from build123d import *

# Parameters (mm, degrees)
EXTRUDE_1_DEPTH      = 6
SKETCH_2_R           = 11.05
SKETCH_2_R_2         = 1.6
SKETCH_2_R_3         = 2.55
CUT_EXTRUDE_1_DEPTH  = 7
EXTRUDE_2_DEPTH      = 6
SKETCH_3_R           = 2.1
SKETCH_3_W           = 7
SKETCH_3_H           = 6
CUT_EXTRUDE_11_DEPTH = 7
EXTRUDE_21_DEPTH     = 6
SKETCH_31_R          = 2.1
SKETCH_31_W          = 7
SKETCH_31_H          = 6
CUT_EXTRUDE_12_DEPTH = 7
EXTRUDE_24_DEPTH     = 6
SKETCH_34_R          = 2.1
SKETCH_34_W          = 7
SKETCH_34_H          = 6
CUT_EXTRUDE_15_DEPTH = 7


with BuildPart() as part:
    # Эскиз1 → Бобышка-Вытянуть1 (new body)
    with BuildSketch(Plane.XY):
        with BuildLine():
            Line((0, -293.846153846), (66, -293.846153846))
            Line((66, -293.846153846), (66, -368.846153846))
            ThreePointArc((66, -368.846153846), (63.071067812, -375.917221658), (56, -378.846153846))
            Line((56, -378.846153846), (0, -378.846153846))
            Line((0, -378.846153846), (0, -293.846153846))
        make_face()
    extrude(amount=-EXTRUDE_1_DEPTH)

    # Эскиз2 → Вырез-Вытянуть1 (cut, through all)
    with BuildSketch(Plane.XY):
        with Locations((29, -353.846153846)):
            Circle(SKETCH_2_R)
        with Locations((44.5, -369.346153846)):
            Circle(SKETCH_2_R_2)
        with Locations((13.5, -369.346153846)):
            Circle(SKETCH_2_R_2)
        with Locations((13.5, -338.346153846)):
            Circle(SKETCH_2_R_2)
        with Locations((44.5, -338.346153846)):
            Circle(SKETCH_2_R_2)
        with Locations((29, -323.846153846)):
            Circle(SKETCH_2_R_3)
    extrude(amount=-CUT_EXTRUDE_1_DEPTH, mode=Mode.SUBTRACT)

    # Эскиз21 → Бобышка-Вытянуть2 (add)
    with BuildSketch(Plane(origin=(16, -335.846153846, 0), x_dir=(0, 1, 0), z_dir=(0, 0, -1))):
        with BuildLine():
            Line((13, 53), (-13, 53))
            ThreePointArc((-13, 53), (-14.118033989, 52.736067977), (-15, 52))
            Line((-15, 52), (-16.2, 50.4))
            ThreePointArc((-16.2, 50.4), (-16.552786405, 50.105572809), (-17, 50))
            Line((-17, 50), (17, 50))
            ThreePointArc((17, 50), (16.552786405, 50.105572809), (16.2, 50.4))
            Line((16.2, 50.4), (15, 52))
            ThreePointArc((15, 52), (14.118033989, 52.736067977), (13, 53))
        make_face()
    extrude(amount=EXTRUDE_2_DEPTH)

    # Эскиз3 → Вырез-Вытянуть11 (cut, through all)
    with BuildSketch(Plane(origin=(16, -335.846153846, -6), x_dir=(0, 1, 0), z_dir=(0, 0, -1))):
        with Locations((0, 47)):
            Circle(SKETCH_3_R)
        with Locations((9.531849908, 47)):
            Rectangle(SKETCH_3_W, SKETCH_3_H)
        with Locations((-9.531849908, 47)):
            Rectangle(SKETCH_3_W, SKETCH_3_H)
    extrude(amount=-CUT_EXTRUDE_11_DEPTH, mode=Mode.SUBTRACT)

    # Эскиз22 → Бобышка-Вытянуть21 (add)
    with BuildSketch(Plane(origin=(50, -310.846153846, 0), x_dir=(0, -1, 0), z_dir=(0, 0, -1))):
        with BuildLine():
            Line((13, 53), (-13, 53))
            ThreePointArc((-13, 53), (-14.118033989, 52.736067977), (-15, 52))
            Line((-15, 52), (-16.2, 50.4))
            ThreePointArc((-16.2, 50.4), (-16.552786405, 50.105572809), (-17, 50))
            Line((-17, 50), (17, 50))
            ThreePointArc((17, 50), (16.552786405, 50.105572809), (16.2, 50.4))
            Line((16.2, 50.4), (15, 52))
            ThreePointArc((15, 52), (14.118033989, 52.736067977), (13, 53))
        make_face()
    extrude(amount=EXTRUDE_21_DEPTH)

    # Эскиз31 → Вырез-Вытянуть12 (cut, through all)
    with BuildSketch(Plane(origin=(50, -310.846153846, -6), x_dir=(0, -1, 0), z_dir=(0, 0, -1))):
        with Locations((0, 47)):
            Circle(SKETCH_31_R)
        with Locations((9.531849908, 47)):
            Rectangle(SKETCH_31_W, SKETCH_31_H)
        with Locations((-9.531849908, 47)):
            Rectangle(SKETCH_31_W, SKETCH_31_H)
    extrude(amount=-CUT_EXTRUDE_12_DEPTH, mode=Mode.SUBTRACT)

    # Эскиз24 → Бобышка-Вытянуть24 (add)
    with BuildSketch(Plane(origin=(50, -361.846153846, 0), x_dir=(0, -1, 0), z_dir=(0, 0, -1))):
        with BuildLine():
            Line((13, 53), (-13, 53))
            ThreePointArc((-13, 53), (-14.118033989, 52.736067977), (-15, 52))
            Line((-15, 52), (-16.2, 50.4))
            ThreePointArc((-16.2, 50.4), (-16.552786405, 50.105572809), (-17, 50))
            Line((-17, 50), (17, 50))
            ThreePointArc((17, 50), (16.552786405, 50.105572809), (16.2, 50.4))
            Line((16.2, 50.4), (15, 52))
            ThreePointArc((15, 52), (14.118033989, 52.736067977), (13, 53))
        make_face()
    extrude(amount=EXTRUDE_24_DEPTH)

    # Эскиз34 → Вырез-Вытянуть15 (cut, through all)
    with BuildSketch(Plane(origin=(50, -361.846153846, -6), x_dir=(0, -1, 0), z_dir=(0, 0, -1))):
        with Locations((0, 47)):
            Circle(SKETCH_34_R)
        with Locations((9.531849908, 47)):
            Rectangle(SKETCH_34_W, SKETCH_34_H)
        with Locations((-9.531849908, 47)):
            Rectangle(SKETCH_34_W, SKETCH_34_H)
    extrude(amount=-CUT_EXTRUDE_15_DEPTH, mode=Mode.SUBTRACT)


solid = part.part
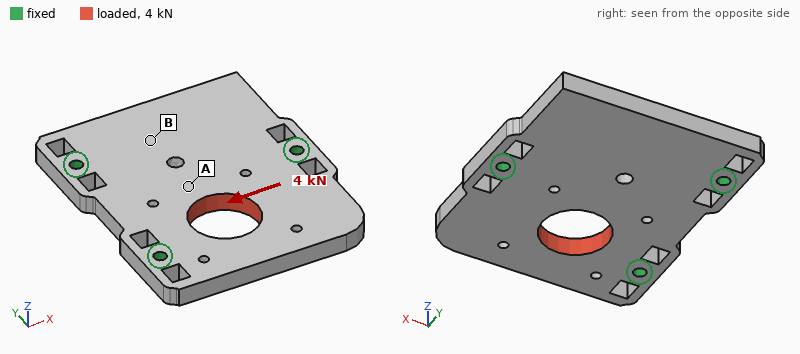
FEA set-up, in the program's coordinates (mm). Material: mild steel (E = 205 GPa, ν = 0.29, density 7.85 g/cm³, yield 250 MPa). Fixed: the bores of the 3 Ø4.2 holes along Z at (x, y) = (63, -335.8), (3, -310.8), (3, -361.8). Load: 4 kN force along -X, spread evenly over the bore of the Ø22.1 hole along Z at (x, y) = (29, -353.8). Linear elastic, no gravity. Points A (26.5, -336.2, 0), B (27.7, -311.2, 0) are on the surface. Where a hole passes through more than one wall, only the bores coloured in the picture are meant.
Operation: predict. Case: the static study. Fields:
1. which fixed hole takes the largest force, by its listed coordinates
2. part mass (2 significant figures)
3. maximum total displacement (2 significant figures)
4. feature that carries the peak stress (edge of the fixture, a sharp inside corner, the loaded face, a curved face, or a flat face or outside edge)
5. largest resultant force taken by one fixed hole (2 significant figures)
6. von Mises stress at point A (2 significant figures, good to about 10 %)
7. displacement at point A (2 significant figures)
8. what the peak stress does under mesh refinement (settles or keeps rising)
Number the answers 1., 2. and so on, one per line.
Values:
1. (3, -361.8)
2. 240 g
3. 3.3 µm
4. edge of the fixture
5. 2.0 kN
6. 7.9 MPa
7. 1.6 µm
8. keeps rising
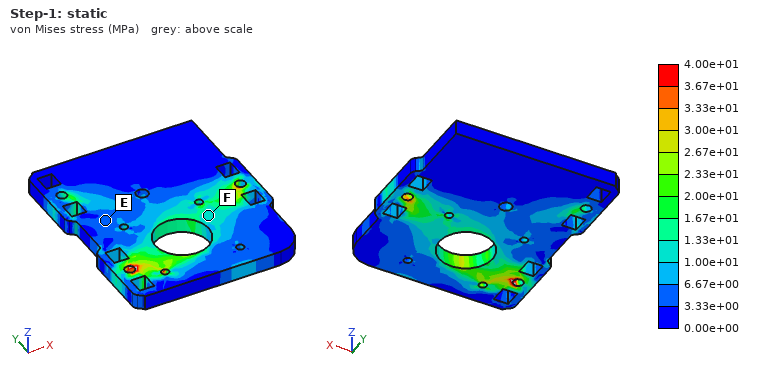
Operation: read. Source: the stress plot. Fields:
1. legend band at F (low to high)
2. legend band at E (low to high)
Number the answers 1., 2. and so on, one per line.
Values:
1. 1.00e+01 to 1.33e+01 MPa
2. 3.33e+00 to 6.67e+00 MPa
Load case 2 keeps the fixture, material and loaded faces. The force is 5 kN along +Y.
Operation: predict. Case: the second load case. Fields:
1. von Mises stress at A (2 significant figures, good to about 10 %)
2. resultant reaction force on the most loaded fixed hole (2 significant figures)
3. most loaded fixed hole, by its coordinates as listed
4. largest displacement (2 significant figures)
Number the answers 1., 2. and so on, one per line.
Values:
1. 12 MPa
2. 2.1 kN
3. (63, -335.8)
4. 5.2 µm
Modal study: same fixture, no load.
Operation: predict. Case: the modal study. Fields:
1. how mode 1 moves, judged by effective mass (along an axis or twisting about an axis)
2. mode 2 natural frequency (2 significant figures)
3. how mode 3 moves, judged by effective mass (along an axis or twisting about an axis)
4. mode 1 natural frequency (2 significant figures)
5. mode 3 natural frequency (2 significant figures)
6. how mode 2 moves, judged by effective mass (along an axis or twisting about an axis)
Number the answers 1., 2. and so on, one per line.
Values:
1. twisting about X
2. 3400 Hz
3. along Z
4. 2900 Hz
5. 6800 Hz
6. along Z
